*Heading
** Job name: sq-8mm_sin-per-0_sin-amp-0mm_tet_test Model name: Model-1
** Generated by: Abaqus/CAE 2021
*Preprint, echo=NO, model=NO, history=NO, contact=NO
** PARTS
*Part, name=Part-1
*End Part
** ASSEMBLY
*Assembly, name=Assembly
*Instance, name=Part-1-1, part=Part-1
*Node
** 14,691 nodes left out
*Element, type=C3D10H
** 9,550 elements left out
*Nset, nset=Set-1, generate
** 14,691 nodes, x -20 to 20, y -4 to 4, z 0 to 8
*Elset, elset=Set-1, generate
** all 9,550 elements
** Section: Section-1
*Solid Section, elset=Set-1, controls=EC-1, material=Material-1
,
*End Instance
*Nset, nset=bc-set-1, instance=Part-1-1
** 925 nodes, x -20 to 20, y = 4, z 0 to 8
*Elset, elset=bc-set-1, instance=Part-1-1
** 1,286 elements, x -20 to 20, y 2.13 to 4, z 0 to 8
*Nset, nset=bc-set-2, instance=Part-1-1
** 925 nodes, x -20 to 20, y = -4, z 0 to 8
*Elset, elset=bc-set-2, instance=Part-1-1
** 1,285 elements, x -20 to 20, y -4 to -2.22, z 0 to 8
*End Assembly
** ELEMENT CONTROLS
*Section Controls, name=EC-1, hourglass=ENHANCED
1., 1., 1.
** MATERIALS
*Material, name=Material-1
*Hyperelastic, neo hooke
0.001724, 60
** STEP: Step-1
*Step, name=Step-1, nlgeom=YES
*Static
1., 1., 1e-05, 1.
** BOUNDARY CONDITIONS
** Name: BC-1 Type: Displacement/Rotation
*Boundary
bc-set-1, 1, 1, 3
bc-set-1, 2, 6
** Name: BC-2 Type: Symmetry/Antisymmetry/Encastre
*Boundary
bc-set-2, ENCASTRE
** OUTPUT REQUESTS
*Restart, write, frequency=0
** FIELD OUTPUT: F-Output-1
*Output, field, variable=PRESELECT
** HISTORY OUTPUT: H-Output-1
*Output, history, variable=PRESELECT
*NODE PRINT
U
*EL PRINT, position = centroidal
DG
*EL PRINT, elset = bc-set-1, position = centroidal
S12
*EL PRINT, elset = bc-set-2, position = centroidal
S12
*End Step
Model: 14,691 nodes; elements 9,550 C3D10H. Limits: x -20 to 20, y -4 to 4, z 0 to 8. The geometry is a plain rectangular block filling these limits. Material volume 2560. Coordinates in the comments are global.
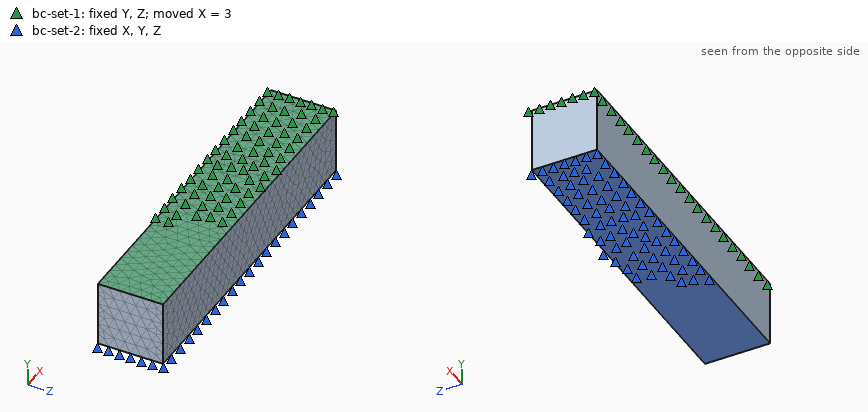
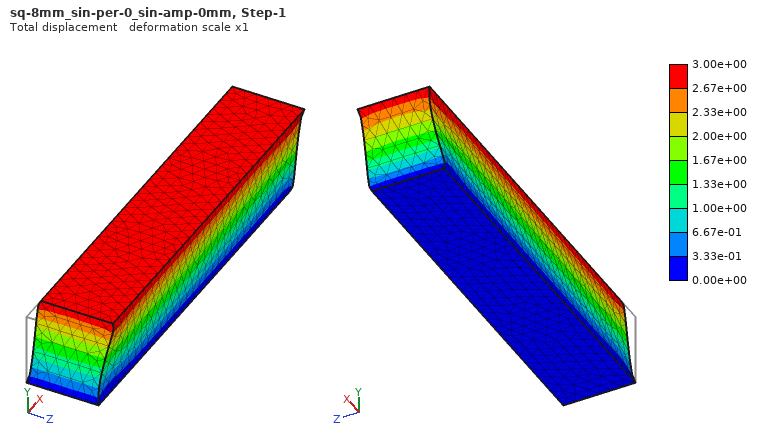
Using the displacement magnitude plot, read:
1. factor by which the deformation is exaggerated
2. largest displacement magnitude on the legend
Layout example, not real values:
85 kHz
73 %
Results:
1
3.00e+00
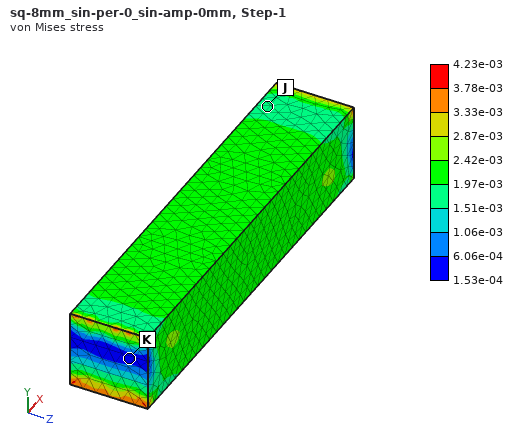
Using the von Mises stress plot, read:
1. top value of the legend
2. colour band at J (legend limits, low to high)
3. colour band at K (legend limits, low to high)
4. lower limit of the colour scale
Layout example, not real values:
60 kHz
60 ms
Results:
4.23e-03
1.51e-03 to 1.97e-03
1.53e-04 to 6.06e-04
1.53e-04
